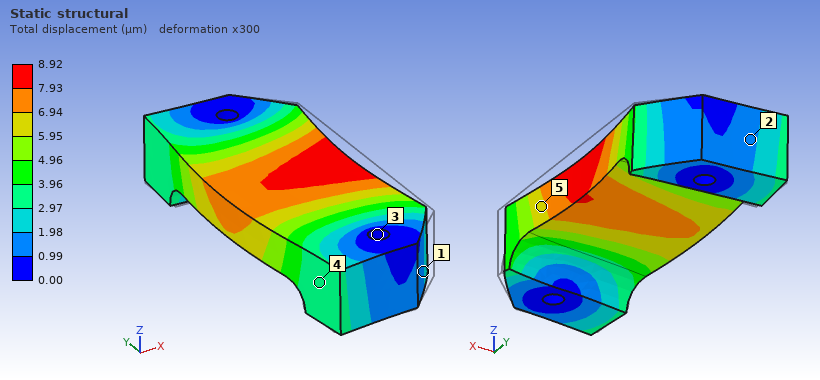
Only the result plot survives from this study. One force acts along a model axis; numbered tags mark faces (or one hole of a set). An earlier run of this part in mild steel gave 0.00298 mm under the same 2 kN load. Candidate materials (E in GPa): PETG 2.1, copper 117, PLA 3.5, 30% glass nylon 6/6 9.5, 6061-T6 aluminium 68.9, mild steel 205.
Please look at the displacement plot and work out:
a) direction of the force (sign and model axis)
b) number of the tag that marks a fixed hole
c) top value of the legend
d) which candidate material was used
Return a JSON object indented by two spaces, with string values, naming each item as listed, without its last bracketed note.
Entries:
{
  "direction of the force": "-X",
  "number of the tag that marks a fixed hole": "3",
  "top value of the legend": "8.92 µm",
  "which candidate material was used": "6061-T6 aluminium"
}
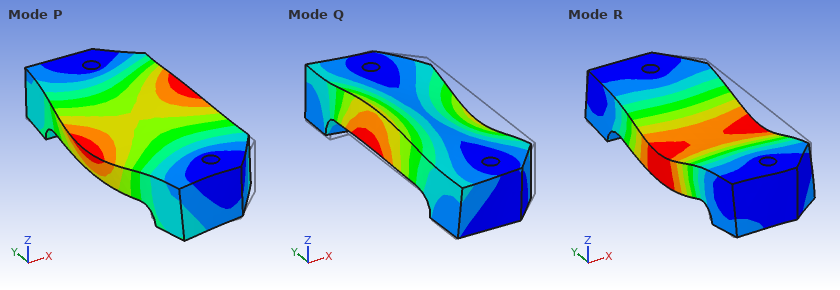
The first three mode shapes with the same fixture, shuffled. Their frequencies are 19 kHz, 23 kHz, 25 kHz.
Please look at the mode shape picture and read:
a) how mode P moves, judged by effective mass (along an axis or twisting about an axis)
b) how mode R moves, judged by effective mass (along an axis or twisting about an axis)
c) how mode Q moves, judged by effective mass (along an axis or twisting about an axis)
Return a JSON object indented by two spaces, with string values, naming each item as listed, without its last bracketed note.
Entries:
{
  "how mode P moves, judged by effective mass": "along X",
  "how mode R moves, judged by effective mass": "along Z",
  "how mode Q moves, judged by effective mass": "along X"
}
